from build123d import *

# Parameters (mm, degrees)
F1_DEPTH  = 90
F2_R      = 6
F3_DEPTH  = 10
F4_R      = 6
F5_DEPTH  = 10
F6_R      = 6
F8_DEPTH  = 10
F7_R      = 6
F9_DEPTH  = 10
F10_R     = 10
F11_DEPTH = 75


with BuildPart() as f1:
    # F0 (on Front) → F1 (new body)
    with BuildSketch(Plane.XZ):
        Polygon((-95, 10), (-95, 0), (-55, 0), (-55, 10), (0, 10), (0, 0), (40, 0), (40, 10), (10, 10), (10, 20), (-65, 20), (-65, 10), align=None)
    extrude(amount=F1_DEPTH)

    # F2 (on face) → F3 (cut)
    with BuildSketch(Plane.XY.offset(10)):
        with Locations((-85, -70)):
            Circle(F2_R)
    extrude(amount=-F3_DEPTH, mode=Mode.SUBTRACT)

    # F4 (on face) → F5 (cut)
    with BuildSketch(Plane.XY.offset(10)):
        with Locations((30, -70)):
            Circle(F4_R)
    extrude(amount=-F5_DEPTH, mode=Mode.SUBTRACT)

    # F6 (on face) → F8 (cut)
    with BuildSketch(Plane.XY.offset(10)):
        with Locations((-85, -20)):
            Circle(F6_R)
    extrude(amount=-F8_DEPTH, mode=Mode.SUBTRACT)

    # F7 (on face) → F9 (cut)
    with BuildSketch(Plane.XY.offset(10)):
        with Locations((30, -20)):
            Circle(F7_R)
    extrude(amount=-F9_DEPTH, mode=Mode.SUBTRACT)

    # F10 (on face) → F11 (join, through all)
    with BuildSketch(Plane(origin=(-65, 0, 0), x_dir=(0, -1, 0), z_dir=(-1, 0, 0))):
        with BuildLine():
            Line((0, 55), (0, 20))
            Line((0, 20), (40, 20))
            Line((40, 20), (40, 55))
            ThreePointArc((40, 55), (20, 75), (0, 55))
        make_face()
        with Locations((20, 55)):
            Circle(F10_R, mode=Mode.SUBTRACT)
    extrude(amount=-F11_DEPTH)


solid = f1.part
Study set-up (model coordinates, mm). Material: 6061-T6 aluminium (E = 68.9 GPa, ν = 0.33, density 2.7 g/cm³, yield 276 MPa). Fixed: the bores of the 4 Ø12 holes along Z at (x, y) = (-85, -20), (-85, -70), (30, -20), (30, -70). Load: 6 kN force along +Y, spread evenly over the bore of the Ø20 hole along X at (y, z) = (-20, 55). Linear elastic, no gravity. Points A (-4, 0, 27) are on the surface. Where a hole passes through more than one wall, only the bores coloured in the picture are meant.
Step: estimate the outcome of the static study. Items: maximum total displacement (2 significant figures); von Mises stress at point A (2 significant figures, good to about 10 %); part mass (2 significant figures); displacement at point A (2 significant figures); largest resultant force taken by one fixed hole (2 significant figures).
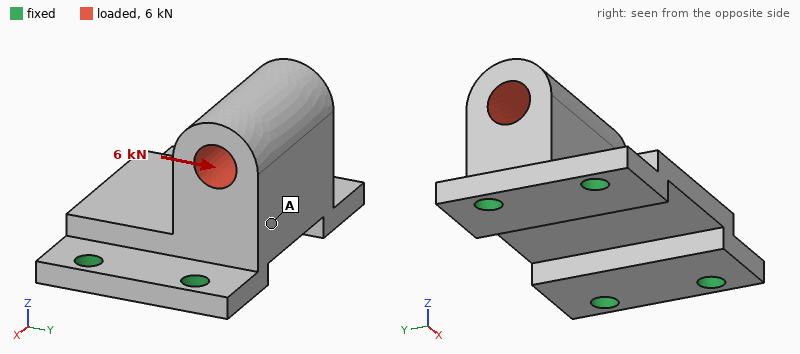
0.14 mm
11 MPa
710 g
0.068 mm
4.9 kN
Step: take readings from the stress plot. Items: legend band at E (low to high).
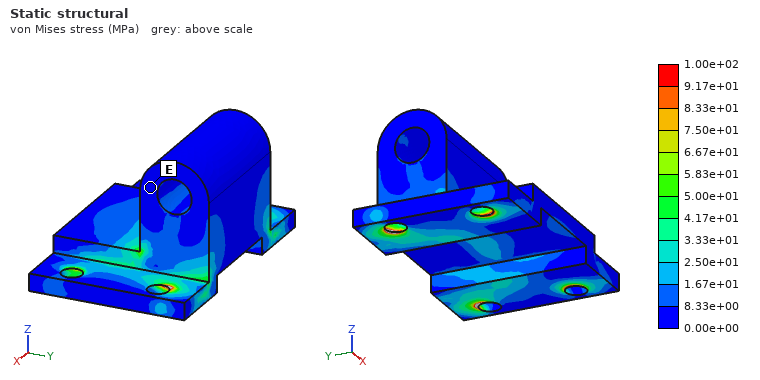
0.00e+00 to 8.33e+00 MPa
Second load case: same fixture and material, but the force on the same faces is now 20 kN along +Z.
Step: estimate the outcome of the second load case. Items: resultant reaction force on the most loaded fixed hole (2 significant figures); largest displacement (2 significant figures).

12 kN
0.13 mm
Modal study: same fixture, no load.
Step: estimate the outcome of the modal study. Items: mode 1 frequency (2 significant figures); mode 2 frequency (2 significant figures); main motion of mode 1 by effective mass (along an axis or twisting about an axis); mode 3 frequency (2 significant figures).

2300 Hz
4200 Hz
along Y
4200 Hz
